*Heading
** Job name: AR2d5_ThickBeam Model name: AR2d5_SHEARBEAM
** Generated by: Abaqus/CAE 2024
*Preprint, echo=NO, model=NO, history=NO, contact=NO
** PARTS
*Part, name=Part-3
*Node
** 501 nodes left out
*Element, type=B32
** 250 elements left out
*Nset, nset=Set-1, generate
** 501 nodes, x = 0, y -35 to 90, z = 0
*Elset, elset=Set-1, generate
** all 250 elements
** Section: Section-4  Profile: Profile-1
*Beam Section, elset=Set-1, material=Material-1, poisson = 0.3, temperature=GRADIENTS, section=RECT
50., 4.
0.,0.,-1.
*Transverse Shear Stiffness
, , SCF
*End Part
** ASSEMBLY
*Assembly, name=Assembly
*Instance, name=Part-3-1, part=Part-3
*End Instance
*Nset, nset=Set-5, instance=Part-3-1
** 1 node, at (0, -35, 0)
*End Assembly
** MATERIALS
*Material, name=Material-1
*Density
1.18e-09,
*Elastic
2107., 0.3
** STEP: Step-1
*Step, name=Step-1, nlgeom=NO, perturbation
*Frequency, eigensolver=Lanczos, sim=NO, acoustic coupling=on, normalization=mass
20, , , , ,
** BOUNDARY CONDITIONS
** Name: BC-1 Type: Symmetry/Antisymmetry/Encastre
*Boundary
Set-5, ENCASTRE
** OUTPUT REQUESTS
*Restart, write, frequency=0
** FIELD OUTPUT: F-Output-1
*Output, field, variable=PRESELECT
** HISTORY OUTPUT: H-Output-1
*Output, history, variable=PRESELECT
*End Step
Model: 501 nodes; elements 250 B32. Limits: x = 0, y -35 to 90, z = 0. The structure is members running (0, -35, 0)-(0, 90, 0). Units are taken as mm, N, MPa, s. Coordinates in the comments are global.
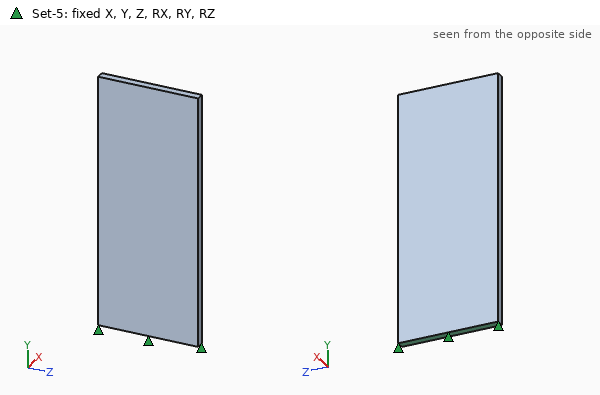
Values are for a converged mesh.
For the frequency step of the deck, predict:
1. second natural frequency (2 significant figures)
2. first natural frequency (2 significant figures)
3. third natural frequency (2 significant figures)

260 Hz
57 Hz
350 Hz
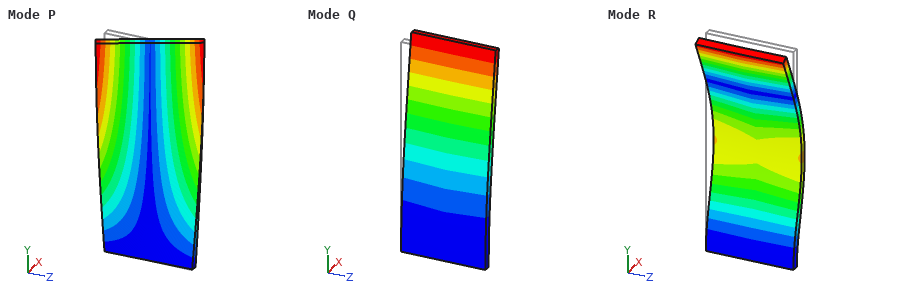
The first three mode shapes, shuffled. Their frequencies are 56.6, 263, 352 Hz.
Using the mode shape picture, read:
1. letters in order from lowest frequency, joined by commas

Q, P, R
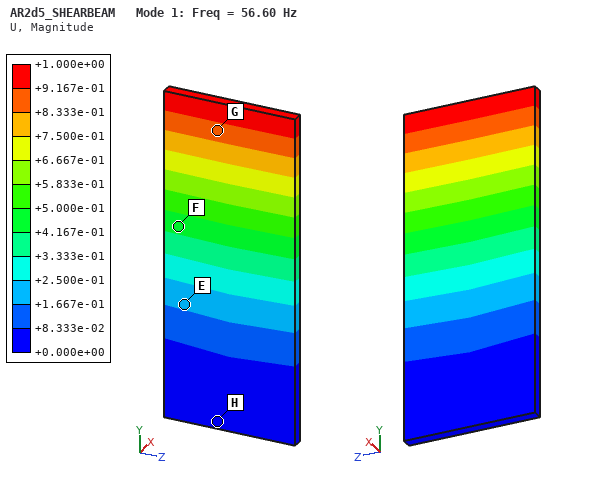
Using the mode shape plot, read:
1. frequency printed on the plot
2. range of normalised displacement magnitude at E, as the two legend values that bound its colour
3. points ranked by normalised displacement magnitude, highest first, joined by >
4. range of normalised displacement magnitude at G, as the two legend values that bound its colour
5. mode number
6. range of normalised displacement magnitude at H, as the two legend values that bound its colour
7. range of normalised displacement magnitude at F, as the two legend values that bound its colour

56.60 Hz
+1.667e-01 to +2.500e-01
G > F > E > H
+8.333e-01 to +9.167e-01
1
+0.000e+00 to +8.333e-02
+4.167e-01 to +5.000e-01
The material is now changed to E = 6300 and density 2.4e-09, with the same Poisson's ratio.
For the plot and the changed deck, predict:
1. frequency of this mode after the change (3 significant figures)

68.6 Hz
